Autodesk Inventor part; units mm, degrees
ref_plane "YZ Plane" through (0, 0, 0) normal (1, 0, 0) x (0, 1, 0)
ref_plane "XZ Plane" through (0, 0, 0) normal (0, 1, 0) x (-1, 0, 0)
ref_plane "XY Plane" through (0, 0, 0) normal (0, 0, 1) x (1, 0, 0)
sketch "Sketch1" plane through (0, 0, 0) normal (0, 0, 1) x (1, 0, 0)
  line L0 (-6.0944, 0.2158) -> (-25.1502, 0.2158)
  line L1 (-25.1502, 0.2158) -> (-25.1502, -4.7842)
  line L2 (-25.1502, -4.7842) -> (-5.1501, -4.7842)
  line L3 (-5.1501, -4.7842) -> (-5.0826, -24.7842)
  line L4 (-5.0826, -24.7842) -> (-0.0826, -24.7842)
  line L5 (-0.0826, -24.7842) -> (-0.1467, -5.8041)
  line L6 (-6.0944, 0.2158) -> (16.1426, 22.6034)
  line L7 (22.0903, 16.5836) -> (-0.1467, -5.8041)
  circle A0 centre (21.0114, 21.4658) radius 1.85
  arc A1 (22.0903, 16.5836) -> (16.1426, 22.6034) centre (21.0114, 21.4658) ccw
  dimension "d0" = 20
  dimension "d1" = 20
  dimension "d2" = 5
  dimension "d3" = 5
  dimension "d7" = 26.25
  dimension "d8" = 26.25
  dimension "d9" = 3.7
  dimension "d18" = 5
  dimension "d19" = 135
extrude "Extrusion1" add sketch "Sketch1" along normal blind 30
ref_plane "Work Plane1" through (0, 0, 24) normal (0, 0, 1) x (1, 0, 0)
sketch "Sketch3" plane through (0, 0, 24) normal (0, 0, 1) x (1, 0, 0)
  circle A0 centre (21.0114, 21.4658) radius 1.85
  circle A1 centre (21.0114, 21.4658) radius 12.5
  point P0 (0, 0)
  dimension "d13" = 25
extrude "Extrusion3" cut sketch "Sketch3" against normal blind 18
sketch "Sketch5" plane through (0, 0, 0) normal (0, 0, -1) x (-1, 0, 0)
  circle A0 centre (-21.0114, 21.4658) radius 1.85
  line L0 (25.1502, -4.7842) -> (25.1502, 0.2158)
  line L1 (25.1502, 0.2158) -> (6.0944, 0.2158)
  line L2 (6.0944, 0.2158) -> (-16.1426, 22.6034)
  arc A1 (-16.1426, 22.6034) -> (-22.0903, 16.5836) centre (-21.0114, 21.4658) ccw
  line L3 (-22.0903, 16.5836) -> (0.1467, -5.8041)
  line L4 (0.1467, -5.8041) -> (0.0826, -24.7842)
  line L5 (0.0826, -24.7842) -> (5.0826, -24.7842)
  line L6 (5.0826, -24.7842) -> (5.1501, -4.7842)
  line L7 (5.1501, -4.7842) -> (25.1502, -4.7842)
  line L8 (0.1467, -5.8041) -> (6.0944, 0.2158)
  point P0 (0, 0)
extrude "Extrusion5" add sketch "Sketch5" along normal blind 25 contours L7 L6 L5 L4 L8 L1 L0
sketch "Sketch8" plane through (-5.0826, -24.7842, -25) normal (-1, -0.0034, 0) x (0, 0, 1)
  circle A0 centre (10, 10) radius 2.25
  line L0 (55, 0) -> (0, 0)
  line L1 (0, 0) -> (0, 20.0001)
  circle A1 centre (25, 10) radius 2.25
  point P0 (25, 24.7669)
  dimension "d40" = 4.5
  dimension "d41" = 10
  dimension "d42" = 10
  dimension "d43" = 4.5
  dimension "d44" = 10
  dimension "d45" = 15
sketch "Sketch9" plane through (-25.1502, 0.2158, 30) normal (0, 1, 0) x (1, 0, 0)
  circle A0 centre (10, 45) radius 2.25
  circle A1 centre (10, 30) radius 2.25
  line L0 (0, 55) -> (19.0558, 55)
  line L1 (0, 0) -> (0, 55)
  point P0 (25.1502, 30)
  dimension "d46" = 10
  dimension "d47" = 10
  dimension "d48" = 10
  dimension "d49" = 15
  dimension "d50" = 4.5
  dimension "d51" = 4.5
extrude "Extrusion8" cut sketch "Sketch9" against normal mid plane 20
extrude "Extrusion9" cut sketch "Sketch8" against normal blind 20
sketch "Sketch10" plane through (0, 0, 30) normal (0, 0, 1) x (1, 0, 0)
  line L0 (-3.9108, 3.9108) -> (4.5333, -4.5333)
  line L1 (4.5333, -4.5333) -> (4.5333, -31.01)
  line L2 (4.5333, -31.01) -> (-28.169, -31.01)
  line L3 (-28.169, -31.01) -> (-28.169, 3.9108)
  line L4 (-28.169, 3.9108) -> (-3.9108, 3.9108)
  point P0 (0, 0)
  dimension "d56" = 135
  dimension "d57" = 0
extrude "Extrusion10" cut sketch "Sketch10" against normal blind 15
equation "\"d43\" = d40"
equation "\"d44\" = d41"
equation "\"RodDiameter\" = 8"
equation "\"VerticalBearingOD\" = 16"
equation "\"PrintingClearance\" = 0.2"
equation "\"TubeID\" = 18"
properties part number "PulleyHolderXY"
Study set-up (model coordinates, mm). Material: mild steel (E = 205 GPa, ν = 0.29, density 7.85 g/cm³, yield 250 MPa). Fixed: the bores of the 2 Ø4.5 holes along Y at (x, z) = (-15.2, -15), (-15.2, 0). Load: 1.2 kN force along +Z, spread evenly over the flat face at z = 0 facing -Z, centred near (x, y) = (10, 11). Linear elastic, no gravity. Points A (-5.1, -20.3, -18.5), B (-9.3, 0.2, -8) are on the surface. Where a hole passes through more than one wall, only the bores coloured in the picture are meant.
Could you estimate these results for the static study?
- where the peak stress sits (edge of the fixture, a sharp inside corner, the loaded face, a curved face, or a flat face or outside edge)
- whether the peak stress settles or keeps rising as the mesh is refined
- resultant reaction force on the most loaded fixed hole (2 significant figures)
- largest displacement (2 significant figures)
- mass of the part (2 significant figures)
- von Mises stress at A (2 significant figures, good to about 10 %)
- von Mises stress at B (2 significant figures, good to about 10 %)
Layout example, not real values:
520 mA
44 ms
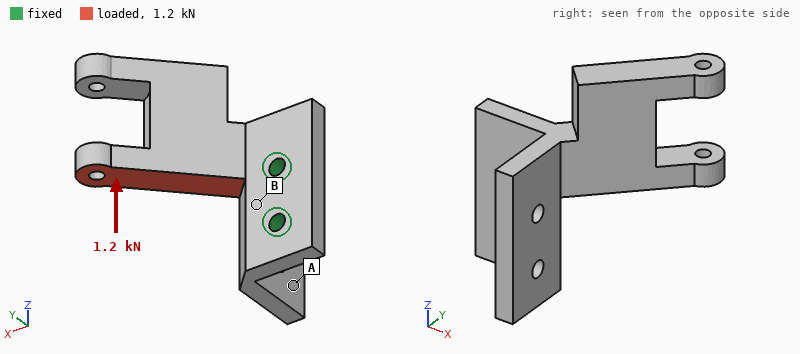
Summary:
edge of the fixture
keeps rising
1.7 kN
0.10 mm
110 g
18 MPa
70 MPa
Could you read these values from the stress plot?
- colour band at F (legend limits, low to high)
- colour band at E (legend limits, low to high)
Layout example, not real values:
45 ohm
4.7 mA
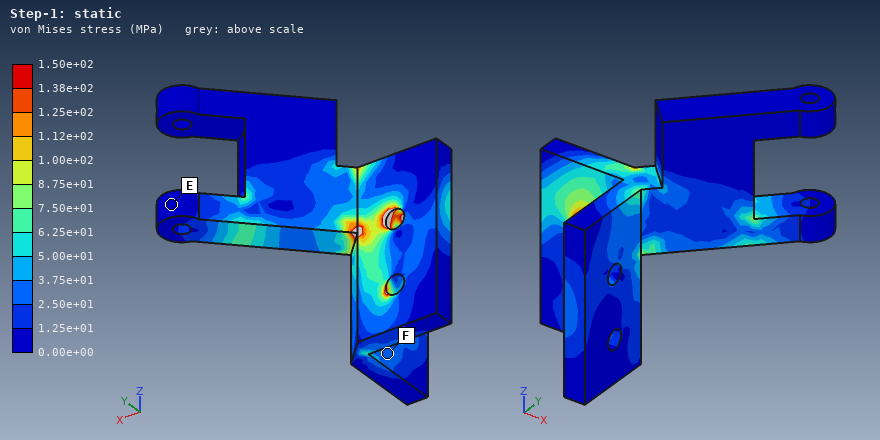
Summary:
2.50e+01 to 3.75e+01 MPa
0.00e+00 to 1.25e+01 MPa
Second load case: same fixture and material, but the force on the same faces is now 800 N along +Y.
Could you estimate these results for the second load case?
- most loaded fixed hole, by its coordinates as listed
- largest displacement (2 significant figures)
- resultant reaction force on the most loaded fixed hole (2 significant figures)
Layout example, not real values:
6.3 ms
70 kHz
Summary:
(-15.2, 0)
0.17 mm
660 N
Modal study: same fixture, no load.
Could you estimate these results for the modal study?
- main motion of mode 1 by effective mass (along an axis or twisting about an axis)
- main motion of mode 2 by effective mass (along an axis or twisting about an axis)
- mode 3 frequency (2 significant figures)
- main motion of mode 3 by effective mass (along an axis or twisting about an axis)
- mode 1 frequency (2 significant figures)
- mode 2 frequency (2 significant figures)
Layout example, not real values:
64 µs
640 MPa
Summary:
along Y
along Z
5100 Hz
along X
1700 Hz
3200 Hz
